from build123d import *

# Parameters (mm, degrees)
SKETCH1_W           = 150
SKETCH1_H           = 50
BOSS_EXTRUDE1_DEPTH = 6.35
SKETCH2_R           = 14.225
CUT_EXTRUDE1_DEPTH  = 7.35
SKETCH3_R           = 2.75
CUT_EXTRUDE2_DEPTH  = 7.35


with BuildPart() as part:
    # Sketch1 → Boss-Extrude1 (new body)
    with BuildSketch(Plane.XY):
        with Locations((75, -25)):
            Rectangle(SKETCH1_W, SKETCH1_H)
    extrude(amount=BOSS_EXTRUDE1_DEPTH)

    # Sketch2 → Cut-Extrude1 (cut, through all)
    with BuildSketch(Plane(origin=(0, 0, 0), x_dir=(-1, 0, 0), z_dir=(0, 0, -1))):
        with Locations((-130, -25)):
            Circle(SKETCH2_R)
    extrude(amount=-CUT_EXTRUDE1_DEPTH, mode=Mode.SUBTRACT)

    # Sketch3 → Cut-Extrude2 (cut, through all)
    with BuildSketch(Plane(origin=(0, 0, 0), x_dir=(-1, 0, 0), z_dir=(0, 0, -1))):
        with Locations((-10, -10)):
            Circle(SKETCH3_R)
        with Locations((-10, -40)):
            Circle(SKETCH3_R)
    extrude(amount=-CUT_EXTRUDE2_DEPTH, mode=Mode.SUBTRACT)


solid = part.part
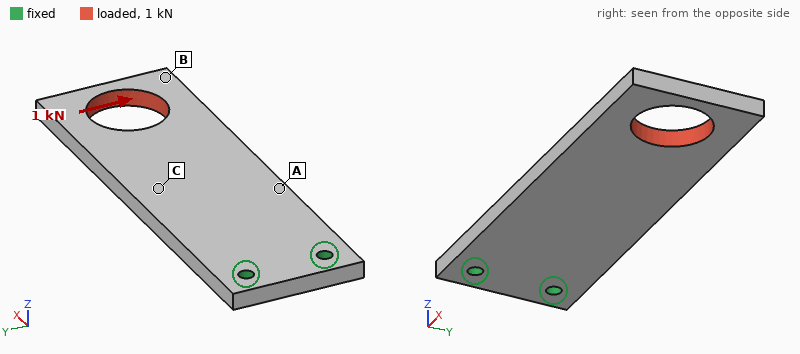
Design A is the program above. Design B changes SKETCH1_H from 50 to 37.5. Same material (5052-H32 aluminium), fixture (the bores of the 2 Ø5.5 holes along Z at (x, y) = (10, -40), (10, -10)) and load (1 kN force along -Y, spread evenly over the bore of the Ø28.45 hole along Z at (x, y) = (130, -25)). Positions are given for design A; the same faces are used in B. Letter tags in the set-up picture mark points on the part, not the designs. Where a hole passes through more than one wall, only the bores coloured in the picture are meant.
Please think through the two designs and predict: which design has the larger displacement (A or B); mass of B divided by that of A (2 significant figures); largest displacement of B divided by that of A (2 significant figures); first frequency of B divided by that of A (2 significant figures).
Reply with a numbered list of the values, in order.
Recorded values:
1. B
2. 0.72
3. 2.1
4. 1.0
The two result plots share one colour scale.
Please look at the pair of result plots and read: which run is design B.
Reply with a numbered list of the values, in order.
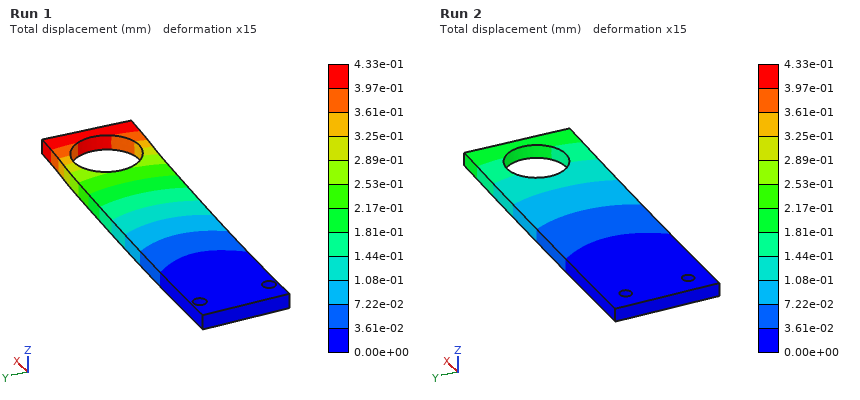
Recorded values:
1. Run 1
